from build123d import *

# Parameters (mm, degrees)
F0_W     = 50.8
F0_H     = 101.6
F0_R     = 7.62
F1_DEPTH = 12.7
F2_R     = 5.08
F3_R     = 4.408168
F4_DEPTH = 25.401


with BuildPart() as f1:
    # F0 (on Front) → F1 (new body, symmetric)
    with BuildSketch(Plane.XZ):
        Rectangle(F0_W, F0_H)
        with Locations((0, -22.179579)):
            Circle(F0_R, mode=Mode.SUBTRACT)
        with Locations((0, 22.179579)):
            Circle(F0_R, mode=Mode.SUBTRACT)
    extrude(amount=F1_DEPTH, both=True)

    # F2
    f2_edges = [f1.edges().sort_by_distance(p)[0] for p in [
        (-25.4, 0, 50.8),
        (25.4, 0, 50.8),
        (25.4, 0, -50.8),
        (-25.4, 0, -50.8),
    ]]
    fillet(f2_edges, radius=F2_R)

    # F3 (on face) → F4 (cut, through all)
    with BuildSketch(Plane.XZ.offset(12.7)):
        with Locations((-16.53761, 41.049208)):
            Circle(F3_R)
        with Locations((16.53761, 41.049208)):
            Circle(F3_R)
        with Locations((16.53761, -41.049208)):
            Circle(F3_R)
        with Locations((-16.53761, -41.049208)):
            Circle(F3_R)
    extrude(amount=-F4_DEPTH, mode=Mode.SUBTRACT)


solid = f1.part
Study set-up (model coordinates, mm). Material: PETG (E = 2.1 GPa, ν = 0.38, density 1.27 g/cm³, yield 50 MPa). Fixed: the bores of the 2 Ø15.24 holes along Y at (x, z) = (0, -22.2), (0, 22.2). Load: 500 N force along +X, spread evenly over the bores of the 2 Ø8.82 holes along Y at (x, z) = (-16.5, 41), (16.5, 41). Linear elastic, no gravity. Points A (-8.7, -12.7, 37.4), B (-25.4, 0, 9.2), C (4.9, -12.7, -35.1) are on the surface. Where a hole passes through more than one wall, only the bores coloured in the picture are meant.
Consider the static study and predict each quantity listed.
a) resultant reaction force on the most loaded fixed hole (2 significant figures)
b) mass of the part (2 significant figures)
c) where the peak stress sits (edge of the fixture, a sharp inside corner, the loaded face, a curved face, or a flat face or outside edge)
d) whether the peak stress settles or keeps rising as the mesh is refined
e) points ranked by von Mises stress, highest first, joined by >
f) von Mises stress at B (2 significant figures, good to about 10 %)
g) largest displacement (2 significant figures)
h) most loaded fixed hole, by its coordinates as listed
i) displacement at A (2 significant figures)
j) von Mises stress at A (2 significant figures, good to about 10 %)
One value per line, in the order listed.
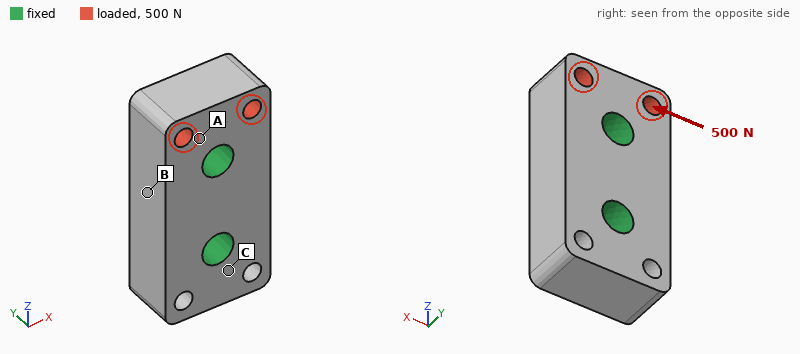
590 N
150 g
edge of the fixture
keeps rising
A > B > C
0.42 MPa
23 µm
(0, 22.2)
10 µm
0.63 MPa
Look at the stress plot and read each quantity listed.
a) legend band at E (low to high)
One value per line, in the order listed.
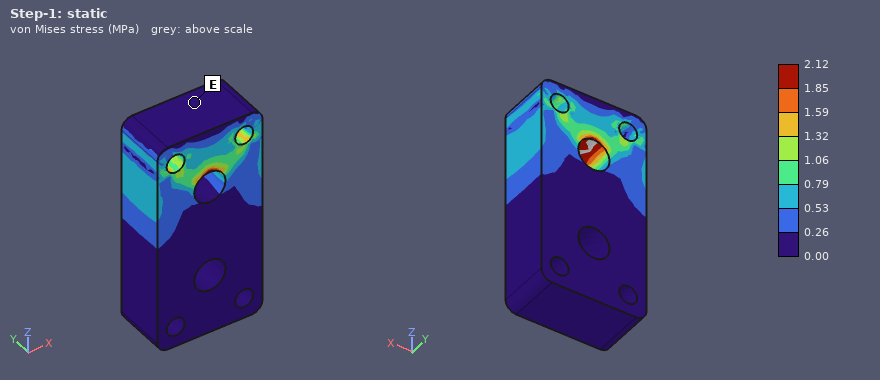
0.00 to 0.26 MPa
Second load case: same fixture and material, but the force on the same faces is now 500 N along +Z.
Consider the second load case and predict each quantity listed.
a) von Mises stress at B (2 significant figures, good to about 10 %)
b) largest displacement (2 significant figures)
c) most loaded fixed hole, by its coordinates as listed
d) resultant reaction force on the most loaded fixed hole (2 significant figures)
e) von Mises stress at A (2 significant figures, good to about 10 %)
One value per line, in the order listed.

0.22 MPa
9.5 µm
(0, 22.2)
410 N
0.63 MPa
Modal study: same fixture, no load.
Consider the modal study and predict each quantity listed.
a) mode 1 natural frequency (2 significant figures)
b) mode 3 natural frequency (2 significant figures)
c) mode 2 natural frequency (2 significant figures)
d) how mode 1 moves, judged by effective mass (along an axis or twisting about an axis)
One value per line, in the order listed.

4500 Hz
4900 Hz
4900 Hz
twisting about Y
